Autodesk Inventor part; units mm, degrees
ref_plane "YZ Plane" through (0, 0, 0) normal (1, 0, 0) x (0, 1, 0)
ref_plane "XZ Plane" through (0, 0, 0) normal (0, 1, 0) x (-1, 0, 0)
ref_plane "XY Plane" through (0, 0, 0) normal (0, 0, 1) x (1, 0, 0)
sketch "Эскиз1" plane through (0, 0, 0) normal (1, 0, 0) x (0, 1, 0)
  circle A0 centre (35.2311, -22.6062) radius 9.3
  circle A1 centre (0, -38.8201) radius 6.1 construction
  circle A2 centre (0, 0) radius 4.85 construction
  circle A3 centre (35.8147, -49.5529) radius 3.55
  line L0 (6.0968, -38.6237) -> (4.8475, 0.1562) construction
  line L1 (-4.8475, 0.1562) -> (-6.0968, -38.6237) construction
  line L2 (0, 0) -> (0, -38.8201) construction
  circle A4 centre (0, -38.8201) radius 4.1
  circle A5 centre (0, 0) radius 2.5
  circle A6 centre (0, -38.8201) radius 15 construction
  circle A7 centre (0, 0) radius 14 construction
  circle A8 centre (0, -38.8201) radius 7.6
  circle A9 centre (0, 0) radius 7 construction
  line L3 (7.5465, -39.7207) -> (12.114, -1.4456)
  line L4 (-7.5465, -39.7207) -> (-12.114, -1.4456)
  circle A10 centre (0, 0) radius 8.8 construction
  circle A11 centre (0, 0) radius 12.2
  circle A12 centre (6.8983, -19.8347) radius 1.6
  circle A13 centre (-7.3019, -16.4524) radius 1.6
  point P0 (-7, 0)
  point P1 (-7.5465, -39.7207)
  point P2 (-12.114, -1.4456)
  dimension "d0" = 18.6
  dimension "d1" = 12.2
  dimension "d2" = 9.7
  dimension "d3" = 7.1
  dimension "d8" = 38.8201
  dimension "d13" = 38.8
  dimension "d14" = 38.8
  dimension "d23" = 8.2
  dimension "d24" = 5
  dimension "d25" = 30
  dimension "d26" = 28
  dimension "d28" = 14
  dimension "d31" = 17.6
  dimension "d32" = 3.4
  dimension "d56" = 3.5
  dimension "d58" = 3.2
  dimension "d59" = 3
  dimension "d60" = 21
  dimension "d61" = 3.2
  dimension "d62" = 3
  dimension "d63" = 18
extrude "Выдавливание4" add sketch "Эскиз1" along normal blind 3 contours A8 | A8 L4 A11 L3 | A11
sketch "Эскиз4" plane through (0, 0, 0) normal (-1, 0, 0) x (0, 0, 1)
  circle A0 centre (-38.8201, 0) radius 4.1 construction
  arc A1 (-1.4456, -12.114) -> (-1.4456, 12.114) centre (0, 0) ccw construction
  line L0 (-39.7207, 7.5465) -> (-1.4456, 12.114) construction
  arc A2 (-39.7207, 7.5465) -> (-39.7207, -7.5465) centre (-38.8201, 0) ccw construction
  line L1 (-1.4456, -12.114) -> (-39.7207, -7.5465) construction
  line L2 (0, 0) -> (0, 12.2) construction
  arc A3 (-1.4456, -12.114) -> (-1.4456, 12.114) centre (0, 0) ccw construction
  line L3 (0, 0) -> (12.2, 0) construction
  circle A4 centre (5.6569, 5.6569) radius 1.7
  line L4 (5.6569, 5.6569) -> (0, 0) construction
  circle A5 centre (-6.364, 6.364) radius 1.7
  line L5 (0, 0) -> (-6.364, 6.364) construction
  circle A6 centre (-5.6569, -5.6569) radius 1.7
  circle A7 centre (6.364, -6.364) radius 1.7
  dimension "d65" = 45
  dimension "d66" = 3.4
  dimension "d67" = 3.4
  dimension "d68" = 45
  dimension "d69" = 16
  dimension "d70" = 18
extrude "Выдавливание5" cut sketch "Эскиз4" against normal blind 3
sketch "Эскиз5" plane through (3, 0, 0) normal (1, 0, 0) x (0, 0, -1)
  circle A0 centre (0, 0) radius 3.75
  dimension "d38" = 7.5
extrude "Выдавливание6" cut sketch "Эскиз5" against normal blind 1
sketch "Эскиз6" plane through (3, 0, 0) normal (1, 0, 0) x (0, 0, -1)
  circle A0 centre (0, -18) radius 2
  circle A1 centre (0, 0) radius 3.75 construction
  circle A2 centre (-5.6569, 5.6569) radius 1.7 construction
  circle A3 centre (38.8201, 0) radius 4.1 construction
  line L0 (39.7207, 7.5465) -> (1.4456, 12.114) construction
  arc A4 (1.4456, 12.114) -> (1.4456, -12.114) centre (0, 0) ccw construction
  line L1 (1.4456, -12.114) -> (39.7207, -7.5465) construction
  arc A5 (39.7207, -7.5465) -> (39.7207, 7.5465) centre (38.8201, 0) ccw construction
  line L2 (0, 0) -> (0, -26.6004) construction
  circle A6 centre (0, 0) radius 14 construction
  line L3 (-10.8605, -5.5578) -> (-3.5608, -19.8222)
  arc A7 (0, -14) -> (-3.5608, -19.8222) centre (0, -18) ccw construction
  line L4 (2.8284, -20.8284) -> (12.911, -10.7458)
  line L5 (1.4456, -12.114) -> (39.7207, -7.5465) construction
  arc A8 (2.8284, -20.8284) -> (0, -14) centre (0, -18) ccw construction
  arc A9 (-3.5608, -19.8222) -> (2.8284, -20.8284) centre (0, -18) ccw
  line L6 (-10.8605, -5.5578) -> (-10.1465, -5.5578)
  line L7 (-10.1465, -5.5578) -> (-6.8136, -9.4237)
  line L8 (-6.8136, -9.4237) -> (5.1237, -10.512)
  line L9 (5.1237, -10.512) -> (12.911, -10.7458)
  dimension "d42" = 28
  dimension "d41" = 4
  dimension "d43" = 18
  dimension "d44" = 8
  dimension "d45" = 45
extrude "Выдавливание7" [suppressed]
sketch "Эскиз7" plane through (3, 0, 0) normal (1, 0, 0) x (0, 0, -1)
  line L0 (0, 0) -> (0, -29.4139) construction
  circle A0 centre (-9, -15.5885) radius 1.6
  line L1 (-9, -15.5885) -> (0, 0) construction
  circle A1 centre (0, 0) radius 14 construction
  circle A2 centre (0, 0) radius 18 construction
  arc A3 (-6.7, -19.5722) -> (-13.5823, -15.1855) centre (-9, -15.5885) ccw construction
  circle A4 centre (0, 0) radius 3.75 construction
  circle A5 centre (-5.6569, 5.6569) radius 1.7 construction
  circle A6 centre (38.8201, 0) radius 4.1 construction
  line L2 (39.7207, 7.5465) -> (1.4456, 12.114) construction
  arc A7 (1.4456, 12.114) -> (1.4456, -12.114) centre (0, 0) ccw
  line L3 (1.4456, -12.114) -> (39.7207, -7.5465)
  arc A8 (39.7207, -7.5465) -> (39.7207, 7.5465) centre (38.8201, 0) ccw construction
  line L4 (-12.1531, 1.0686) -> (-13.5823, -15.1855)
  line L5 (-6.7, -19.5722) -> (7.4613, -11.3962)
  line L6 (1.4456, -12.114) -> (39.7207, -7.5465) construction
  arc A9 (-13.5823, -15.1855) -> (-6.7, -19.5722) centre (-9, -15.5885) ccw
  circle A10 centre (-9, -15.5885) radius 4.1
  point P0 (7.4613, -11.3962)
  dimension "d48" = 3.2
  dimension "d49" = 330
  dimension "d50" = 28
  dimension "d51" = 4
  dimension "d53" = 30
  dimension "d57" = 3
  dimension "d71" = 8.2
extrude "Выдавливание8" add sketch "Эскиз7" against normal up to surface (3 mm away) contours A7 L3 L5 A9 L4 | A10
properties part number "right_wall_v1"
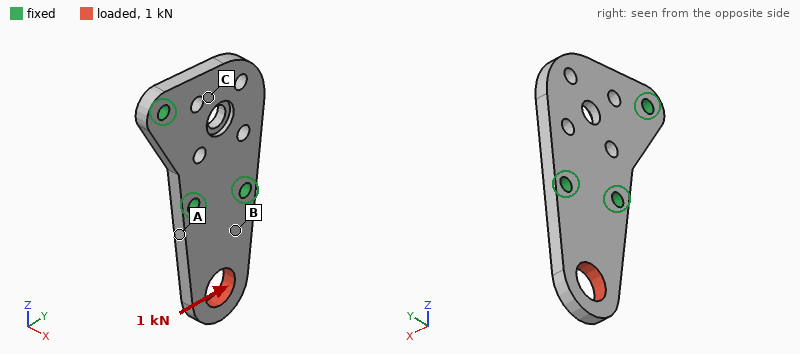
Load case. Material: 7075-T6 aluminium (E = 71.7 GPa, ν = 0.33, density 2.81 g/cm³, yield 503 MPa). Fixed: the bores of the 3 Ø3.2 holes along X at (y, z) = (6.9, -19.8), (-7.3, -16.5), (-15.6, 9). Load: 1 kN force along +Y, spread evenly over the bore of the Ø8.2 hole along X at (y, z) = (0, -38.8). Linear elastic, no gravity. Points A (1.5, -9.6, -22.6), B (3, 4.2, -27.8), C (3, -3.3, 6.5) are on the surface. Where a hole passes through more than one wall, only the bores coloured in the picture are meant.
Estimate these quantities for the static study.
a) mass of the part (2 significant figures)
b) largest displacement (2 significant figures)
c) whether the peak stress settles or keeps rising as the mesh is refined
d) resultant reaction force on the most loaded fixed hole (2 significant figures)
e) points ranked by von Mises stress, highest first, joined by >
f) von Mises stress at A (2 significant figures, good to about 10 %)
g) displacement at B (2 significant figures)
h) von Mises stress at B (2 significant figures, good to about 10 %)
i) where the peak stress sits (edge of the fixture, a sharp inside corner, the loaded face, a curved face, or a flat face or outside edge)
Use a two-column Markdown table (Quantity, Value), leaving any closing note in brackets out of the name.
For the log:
| Quantity | Value |
|---|---|
| mass of the part | 9.2 g |
| largest displacement | 66 µm |
| whether the peak stress settles or keeps rising as the mesh is refined | keeps rising |
| resultant reaction force on the most loaded fixed hole | 1.4 kN |
| points ranked by von Mises stress, highest first, joined by > | A > B > C |
| von Mises stress at A | 82 MPa |
| displacement at B | 11 µm |
| von Mises stress at B | 43 MPa |
| where the peak stress sits | edge of the fixture |
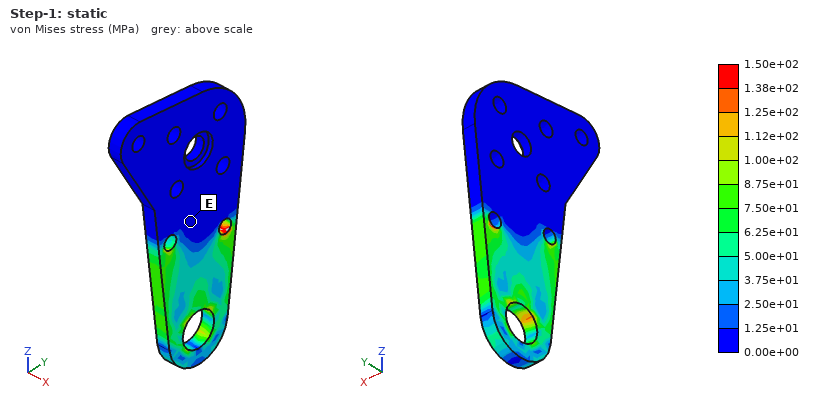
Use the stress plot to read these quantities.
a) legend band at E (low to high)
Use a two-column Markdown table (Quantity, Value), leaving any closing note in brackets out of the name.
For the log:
| Quantity | Value |
|---|---|
| legend band at E | 0.00e+00 to 1.25e+01 MPa |
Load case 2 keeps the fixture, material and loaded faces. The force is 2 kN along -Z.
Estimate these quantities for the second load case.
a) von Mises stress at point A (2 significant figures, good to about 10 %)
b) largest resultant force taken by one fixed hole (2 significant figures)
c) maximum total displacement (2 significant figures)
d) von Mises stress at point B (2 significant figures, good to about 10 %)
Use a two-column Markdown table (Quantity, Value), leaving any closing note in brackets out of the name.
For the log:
| Quantity | Value |
|---|---|
| von Mises stress at point A | 42 MPa |
| largest resultant force taken by one fixed hole | 1.0 kN |
| maximum total displacement | 23 µm |
| von Mises stress at point B | 36 MPa |
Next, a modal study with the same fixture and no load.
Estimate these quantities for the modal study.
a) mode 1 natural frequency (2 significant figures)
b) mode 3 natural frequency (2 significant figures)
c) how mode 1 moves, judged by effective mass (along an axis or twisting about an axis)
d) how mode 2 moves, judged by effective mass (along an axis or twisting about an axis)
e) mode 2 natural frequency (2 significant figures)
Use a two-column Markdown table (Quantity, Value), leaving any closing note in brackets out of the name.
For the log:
| Quantity | Value |
|---|---|
| mode 1 natural frequency | 4500 Hz |
| mode 3 natural frequency | 14 kHz |
| how mode 1 moves, judged by effective mass | along X |
| how mode 2 moves, judged by effective mass | along X |
| mode 2 natural frequency | 6300 Hz |
